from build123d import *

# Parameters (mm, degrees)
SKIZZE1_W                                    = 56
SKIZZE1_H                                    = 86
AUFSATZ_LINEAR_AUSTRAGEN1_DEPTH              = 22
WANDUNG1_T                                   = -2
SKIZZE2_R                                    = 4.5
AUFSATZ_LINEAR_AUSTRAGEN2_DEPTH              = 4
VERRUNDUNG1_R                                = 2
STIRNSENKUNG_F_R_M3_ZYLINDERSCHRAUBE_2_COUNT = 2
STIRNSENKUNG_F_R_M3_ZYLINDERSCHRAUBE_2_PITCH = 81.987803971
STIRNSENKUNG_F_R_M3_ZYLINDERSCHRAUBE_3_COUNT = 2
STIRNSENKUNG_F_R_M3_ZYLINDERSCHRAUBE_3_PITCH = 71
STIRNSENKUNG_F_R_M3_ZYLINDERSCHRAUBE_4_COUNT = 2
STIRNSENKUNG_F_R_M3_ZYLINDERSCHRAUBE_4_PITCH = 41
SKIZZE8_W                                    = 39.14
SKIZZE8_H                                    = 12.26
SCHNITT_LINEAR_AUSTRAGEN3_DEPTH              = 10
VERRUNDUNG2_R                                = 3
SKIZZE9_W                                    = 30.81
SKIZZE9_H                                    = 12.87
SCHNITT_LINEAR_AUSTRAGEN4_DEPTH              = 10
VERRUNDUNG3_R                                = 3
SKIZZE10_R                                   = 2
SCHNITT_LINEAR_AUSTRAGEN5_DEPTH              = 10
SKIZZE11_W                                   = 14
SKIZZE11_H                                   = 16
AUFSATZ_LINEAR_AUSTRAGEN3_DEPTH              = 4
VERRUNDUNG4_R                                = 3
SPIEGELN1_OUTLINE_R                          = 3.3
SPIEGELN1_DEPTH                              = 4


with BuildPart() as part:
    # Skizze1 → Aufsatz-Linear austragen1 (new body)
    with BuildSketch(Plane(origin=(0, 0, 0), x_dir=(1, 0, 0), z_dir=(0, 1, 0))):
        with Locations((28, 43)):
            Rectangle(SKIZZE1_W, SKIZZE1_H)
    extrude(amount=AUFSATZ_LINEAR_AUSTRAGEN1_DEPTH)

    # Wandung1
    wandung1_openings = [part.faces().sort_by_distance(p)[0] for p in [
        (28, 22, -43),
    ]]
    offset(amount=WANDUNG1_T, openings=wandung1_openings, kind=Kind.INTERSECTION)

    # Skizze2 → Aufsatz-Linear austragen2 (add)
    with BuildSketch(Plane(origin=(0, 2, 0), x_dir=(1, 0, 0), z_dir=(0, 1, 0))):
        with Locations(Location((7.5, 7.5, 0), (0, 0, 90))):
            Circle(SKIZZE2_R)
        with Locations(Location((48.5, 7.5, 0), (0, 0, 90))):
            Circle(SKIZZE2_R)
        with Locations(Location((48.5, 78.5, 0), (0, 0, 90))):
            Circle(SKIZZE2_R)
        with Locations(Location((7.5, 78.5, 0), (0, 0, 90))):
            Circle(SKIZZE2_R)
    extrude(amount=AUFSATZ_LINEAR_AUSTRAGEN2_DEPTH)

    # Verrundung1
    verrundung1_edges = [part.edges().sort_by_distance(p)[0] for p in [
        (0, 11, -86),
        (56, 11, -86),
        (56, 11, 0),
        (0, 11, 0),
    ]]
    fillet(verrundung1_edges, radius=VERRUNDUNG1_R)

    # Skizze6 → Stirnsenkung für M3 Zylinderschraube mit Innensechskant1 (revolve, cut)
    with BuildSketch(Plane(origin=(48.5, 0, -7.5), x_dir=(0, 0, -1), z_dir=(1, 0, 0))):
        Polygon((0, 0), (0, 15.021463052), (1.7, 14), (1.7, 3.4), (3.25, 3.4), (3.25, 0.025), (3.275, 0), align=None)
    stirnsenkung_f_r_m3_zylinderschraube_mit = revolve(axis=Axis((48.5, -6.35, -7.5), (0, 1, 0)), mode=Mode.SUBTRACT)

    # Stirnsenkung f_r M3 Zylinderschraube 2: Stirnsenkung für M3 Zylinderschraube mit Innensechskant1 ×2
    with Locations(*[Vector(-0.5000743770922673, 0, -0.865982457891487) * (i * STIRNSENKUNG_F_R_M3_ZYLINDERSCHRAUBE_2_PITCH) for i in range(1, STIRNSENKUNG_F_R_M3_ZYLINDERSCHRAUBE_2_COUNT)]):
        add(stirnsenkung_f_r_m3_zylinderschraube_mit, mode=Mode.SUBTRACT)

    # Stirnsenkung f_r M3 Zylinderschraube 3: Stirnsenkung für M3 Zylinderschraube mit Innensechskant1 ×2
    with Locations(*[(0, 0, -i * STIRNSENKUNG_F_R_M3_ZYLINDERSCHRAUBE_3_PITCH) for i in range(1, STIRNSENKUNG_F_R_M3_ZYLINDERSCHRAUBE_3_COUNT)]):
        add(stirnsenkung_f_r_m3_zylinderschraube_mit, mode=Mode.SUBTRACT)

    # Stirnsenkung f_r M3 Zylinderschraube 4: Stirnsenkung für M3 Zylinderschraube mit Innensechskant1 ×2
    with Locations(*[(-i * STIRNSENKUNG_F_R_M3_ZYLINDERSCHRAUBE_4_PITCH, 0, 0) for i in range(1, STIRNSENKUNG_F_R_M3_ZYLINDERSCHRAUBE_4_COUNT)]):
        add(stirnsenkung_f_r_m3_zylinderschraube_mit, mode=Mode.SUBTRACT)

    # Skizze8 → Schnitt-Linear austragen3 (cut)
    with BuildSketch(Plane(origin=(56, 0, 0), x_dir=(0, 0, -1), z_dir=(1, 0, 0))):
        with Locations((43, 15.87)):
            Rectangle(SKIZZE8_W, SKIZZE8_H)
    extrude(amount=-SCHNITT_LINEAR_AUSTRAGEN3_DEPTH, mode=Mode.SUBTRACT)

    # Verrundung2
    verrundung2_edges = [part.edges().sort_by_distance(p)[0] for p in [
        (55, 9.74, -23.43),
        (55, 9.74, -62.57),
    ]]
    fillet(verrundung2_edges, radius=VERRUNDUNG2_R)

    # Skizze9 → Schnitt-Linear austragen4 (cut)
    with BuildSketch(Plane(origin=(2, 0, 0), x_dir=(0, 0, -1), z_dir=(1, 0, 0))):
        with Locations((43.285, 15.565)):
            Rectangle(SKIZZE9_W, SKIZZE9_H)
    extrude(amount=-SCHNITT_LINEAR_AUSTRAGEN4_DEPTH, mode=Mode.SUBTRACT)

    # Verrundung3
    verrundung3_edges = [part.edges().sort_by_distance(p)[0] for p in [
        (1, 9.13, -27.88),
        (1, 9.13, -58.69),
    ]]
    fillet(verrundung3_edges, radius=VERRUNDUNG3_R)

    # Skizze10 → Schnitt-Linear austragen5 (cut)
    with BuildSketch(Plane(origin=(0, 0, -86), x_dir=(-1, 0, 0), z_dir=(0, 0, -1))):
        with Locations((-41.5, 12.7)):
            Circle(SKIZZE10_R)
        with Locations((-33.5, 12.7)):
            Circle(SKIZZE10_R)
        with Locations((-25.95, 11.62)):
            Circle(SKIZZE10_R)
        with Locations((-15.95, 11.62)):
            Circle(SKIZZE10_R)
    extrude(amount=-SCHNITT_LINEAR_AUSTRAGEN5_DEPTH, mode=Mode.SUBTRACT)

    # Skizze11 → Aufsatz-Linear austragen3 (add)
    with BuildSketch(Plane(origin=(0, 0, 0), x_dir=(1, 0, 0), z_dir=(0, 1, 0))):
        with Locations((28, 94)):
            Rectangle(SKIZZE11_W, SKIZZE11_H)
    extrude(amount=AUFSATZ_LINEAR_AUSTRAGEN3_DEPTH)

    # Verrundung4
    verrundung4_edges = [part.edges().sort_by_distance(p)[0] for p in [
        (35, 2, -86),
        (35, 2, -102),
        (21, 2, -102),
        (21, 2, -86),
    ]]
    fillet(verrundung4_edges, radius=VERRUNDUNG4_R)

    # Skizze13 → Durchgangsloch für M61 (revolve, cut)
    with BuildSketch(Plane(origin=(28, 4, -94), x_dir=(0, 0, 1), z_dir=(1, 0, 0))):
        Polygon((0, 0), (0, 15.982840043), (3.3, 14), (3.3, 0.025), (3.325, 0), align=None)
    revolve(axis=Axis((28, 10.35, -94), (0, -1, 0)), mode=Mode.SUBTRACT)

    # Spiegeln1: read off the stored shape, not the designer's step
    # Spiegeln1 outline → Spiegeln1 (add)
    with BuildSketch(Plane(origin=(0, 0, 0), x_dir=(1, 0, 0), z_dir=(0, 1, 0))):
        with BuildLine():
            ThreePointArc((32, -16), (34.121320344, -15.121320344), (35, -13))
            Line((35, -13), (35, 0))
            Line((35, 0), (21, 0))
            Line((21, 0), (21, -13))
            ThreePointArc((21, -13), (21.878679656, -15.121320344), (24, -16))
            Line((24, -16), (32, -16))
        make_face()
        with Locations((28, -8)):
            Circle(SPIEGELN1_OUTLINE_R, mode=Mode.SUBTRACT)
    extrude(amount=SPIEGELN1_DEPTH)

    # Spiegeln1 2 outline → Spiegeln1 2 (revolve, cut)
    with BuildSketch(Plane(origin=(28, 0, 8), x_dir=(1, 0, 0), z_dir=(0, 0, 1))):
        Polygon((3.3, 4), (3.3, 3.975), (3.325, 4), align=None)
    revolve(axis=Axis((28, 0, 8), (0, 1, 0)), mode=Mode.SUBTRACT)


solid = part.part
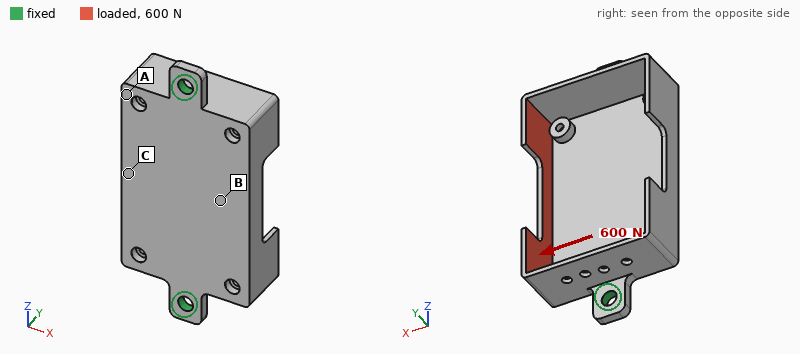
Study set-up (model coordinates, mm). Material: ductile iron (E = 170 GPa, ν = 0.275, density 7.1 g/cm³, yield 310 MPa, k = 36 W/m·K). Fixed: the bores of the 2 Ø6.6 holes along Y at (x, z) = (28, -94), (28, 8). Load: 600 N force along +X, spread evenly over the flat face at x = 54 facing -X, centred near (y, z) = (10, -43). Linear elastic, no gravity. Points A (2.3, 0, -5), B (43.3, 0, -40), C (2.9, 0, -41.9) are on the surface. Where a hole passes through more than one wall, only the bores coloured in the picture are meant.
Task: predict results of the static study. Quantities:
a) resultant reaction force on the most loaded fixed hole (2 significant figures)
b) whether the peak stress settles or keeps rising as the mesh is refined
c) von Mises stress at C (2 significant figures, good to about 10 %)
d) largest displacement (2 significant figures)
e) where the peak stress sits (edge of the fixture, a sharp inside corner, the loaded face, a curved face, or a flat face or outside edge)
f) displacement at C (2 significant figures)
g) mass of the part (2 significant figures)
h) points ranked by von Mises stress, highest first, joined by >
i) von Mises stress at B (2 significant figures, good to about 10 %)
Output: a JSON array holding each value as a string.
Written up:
["300 N", "keeps rising", "7.8 MPa", "91 µm", "edge of the fixture", "26 µm", "150 g", "B > C > A", "17 MPa"]
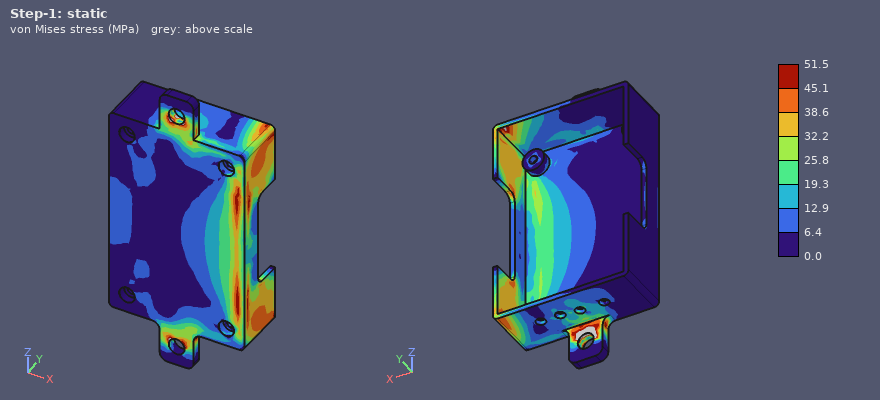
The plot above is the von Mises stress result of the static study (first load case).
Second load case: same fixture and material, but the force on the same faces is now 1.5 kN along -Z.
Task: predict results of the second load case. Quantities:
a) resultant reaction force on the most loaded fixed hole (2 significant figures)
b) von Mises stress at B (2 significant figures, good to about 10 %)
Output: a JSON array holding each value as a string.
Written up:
["880 N", "9.9 MPa"]
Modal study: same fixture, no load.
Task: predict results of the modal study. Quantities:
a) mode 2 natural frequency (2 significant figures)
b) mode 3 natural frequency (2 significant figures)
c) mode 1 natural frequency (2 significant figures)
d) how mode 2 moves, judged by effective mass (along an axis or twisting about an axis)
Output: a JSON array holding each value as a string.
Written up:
["1900 Hz", "2300 Hz", "1500 Hz", "along Y"]
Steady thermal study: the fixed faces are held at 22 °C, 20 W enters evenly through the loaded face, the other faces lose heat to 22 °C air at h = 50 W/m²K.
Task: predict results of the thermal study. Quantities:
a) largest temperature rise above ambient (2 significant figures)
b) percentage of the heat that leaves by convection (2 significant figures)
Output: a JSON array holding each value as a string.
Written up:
["65 K", "81 %"]
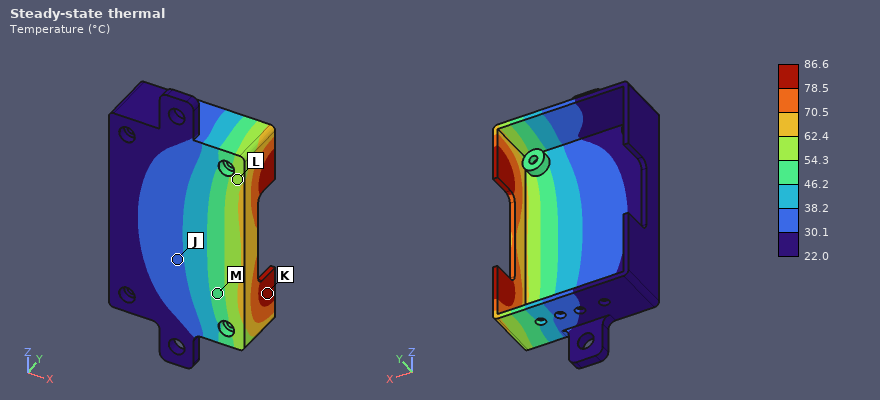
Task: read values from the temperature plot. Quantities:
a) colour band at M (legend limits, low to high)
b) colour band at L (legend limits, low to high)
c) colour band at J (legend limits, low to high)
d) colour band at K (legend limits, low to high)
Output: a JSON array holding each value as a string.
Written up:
["46.2 to 54.3 °C", "54.3 to 62.4 °C", "30.1 to 38.2 °C", "78.5 to 86.6 °C"]
